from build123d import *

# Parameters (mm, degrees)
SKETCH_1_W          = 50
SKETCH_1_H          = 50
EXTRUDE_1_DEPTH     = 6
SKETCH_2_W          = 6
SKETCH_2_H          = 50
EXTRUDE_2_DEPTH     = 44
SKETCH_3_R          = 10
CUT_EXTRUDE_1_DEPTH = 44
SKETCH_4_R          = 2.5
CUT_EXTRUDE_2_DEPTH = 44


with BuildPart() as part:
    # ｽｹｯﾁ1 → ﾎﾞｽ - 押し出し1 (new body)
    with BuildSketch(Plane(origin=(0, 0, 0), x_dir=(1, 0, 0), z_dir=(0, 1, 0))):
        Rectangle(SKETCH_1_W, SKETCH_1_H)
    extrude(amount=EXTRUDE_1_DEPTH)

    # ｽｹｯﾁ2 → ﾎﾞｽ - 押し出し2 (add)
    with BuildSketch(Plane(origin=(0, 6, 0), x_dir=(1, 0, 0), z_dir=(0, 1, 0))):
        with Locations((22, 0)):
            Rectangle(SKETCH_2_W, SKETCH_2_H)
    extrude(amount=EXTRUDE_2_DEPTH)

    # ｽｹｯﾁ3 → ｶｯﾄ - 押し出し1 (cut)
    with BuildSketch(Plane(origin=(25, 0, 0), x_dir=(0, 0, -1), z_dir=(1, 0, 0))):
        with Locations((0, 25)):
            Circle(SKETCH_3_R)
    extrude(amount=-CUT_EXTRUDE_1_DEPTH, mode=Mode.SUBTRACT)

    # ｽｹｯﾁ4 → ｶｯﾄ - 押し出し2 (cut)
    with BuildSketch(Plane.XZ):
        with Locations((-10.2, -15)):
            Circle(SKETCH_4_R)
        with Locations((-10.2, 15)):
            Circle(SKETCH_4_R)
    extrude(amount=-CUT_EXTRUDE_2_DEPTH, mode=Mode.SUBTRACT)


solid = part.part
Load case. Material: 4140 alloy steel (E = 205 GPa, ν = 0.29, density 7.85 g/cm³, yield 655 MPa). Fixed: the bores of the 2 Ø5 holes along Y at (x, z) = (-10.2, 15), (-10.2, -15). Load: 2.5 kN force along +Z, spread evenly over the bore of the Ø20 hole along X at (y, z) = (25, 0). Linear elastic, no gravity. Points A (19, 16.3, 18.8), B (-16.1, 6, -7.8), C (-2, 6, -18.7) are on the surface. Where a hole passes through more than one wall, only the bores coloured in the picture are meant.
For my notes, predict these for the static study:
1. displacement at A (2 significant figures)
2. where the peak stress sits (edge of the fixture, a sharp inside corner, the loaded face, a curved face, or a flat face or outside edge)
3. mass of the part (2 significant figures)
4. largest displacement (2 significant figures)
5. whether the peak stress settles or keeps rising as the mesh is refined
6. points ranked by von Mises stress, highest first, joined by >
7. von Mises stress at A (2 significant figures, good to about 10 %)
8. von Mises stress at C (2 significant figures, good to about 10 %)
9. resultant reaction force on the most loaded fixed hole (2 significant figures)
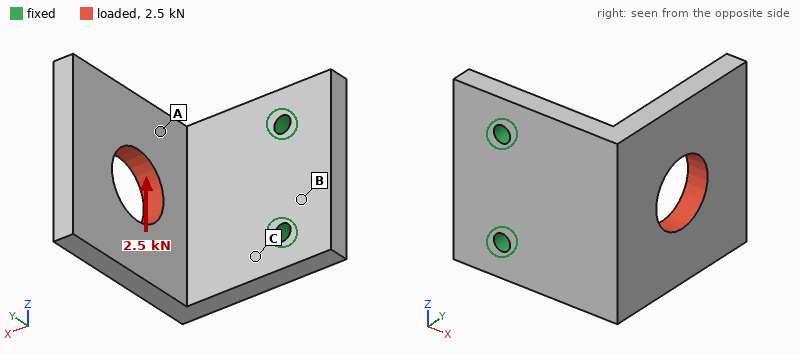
0.082 mm
edge of the fixture
200 g
0.19 mm
keeps rising
C > A > B
52 MPa
97 MPa
3.1 kN
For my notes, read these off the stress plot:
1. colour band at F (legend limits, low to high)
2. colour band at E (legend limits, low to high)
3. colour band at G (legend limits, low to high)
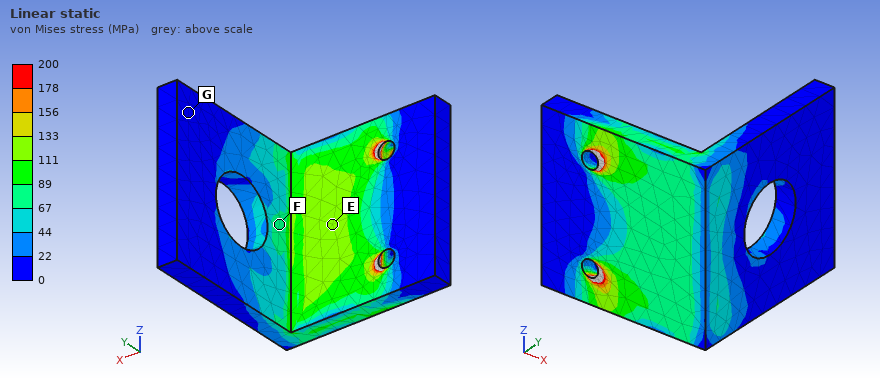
67 to 89 MPa
111 to 133 MPa
0 to 22 MPa
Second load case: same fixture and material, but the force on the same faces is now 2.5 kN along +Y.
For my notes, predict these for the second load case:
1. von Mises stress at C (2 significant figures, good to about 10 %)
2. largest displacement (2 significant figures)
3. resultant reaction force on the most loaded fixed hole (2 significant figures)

200 MPa
0.38 mm
1.3 kN
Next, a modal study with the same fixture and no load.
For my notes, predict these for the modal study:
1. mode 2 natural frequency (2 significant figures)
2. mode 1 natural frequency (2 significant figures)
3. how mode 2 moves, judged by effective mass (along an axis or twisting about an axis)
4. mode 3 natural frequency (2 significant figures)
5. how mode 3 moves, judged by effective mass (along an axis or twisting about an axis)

2000 Hz
1100 Hz
along Z
3000 Hz
along Y
